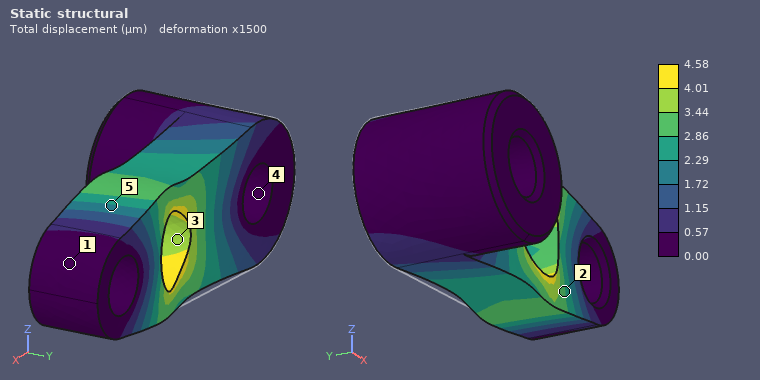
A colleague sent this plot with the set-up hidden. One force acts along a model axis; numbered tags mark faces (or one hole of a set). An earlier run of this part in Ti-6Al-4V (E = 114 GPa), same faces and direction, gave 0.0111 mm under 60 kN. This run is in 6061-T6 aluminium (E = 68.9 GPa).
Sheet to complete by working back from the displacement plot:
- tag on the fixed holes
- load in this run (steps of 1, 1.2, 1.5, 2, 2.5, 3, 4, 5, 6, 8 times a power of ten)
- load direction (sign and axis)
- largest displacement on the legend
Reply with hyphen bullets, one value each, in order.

- 4
- 15 kN
- +X
- 4.58 µm
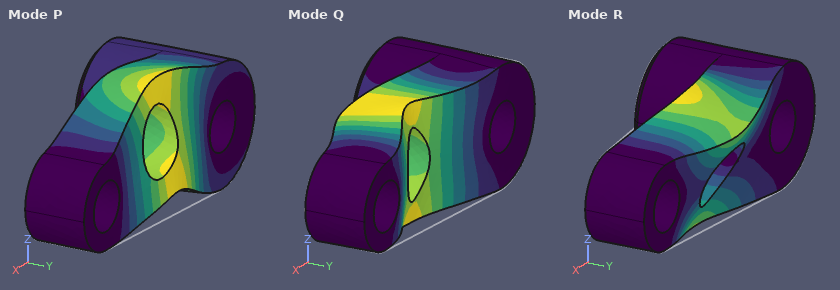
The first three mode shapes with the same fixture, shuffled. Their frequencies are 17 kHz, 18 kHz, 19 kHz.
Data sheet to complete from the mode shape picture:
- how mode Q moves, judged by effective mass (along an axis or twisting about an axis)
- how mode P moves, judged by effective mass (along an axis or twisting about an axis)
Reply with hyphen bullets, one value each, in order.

- along Y
- along Z
